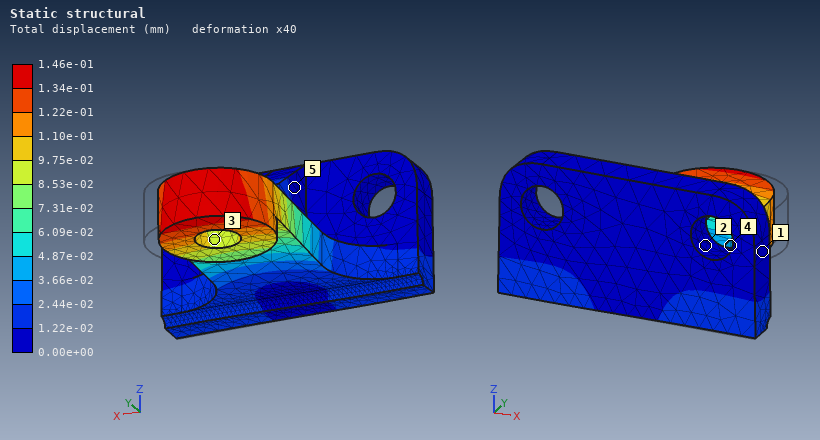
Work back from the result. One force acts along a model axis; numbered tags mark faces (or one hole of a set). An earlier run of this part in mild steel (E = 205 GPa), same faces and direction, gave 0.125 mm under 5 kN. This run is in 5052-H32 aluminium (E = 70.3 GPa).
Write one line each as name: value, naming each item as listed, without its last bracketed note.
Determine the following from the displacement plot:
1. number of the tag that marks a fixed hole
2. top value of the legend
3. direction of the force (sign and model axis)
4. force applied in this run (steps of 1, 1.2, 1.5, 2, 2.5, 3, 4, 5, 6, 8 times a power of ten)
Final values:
number of the tag that marks a fixed hole: 2
top value of the legend: 1.46e-01 mm
direction of the force: -X
force applied in this run: 2 kN
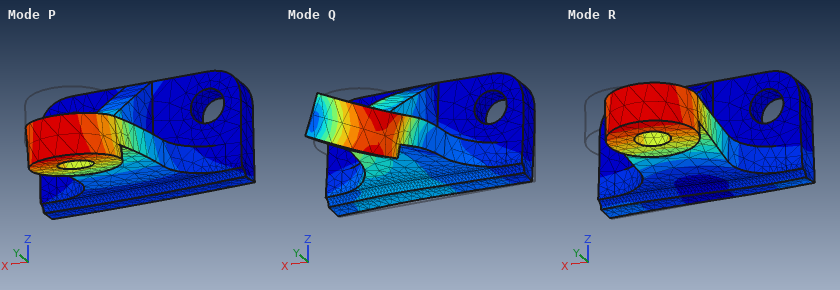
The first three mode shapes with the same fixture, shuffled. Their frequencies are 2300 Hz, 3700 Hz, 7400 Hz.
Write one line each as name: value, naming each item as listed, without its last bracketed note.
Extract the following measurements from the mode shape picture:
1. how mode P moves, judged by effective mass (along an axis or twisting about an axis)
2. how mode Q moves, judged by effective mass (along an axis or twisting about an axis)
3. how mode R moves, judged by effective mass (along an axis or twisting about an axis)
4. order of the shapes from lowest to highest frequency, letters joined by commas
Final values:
how mode P moves, judged by effective mass: along Z
how mode Q moves, judged by effective mass: along Y
how mode R moves, judged by effective mass: along X
order of the shapes from lowest to highest frequency, letters joined by commas: P, R, Q
